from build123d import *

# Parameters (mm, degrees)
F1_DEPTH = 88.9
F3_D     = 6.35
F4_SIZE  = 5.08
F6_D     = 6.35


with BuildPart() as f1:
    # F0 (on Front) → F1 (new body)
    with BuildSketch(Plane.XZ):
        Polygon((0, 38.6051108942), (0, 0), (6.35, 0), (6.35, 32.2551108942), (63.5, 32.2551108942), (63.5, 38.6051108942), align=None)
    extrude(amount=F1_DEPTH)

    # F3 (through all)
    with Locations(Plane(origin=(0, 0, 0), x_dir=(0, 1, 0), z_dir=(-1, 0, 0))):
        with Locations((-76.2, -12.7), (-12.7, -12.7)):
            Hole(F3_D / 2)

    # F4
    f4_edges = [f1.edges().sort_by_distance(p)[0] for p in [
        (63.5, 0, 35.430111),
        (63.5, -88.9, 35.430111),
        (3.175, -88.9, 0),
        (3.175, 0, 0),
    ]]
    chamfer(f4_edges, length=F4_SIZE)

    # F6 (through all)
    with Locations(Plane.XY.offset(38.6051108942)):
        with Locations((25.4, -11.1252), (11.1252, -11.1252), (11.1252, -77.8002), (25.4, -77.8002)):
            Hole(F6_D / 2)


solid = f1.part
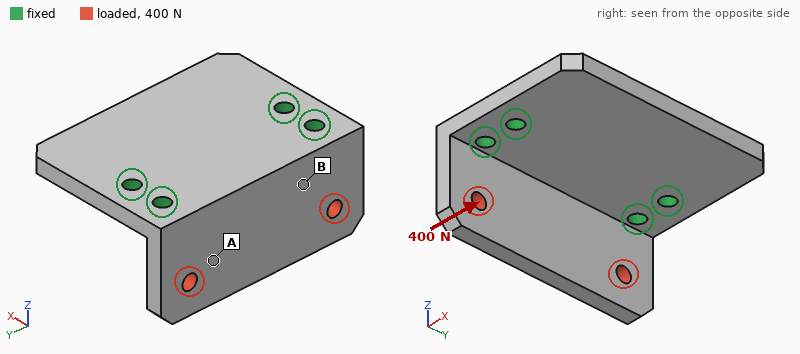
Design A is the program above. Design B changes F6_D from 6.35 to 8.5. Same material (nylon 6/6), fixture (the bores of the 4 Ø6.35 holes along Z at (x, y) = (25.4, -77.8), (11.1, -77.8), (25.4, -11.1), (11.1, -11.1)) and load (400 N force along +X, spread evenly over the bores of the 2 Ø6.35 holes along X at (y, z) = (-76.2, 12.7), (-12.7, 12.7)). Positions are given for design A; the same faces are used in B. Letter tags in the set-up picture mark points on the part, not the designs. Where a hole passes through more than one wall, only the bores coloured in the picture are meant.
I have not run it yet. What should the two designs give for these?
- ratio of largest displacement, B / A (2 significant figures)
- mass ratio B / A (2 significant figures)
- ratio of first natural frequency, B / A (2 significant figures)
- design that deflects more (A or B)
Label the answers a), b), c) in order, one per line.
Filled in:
a) 0.91
b) 0.99
c) 1.1
d) A
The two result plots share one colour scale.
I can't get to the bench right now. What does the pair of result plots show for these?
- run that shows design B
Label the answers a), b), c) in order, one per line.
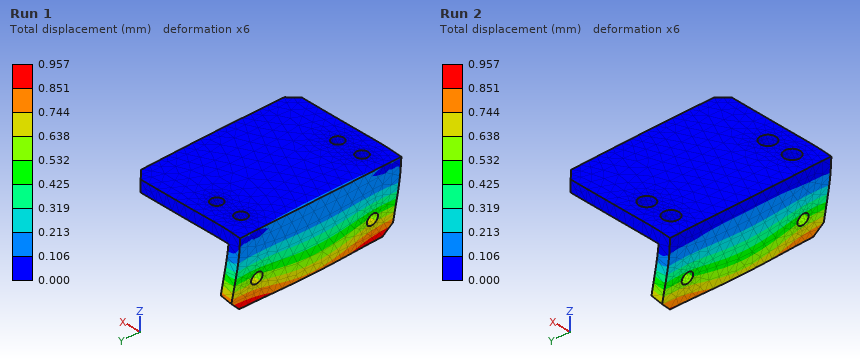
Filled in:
a) Run 2
